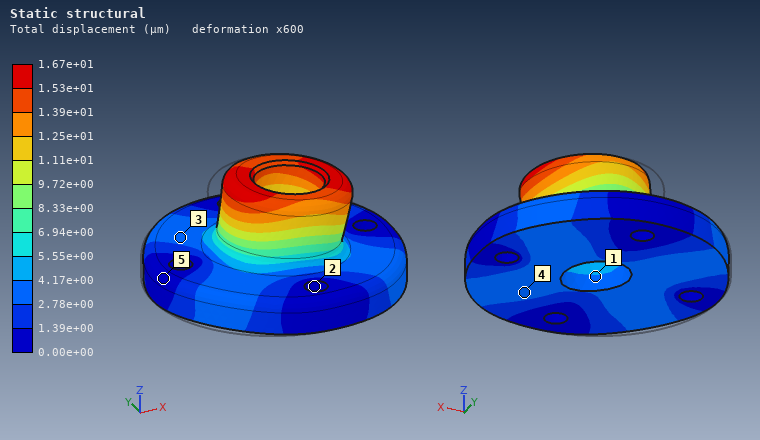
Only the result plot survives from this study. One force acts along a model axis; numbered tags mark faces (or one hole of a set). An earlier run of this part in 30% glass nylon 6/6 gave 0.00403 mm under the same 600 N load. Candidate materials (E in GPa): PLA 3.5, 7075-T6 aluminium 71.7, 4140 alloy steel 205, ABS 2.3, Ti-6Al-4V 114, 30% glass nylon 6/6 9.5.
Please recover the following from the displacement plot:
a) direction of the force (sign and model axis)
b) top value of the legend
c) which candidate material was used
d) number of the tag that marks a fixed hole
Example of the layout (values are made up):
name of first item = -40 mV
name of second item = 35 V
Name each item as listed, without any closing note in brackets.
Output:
direction of the force = +X
top value of the legend = 1.67e+01 µm
which candidate material was used = ABS
number of the tag that marks a fixed hole = 2
